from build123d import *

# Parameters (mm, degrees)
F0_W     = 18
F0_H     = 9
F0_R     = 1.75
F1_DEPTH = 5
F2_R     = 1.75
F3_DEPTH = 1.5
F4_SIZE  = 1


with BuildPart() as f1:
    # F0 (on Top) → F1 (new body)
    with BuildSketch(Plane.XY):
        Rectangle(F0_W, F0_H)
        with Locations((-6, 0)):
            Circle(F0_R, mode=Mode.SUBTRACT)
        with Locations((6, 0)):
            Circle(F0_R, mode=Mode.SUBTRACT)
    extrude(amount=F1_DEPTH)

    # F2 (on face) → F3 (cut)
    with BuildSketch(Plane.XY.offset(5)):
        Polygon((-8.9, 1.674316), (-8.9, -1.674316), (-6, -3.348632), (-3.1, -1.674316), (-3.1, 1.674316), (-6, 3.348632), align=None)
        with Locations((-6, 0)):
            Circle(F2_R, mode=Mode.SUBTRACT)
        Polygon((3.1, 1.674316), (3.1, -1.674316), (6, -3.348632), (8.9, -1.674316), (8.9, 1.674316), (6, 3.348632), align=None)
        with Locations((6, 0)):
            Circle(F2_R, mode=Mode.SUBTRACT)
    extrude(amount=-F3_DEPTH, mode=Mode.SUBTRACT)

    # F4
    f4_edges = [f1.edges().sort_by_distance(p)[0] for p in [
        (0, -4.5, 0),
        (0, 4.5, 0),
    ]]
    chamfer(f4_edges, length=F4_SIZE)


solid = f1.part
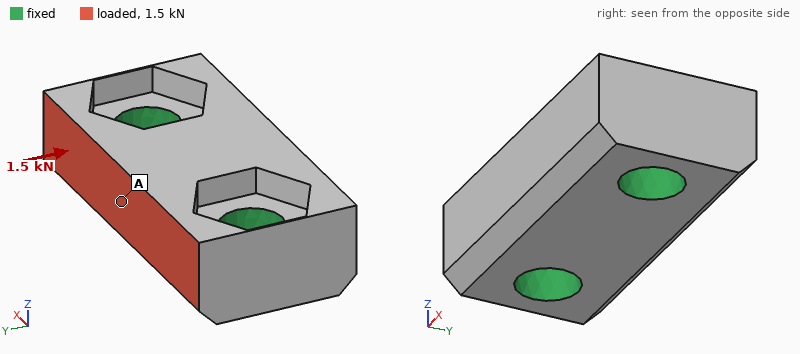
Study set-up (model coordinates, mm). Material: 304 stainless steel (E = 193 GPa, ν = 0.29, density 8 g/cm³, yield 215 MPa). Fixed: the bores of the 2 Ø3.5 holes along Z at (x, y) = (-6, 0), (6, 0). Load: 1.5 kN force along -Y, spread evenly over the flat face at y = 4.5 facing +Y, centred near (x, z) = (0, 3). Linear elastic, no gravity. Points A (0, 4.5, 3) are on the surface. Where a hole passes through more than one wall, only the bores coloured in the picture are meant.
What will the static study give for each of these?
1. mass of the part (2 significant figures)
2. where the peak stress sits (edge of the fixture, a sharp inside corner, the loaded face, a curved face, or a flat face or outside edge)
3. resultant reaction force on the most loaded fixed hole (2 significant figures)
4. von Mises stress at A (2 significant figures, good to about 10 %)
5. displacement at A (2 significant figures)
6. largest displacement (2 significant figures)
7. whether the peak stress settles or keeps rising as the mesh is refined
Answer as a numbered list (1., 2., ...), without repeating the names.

1. 5.1 g
2. edge of the fixture
3. 750 N
4. 17 MPa
5. 1.5 µm
6. 2.2 µm
7. keeps rising
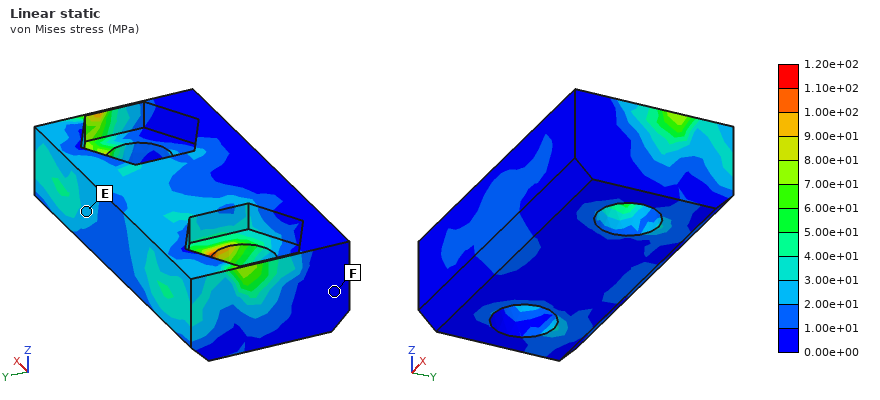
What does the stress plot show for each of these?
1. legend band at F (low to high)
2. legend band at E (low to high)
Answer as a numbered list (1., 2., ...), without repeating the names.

1. 0.00e+00 to 1.00e+01 MPa
2. 2.00e+01 to 3.00e+01 MPa
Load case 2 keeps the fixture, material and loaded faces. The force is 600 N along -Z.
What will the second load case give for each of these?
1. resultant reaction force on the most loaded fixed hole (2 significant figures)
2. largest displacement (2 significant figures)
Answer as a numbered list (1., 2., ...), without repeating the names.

1. 300 N
2. 2.1 µm
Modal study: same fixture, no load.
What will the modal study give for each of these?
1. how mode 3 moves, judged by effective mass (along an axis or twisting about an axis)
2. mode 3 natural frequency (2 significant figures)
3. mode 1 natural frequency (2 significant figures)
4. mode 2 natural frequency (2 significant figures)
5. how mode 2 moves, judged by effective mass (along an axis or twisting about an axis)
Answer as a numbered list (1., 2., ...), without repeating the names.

1. along Y
2. 120 kHz
3. 81 kHz
4. 96 kHz
5. along Z
